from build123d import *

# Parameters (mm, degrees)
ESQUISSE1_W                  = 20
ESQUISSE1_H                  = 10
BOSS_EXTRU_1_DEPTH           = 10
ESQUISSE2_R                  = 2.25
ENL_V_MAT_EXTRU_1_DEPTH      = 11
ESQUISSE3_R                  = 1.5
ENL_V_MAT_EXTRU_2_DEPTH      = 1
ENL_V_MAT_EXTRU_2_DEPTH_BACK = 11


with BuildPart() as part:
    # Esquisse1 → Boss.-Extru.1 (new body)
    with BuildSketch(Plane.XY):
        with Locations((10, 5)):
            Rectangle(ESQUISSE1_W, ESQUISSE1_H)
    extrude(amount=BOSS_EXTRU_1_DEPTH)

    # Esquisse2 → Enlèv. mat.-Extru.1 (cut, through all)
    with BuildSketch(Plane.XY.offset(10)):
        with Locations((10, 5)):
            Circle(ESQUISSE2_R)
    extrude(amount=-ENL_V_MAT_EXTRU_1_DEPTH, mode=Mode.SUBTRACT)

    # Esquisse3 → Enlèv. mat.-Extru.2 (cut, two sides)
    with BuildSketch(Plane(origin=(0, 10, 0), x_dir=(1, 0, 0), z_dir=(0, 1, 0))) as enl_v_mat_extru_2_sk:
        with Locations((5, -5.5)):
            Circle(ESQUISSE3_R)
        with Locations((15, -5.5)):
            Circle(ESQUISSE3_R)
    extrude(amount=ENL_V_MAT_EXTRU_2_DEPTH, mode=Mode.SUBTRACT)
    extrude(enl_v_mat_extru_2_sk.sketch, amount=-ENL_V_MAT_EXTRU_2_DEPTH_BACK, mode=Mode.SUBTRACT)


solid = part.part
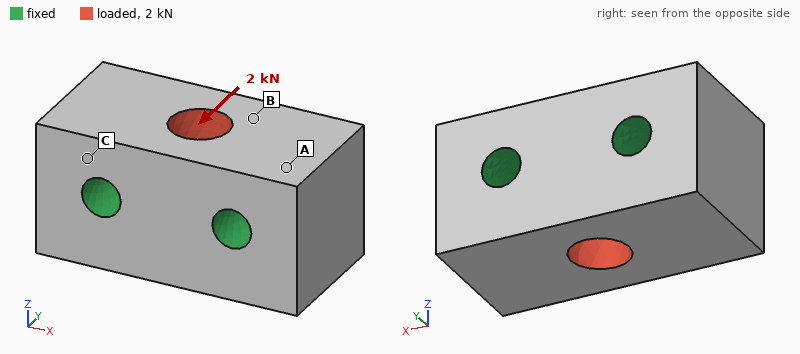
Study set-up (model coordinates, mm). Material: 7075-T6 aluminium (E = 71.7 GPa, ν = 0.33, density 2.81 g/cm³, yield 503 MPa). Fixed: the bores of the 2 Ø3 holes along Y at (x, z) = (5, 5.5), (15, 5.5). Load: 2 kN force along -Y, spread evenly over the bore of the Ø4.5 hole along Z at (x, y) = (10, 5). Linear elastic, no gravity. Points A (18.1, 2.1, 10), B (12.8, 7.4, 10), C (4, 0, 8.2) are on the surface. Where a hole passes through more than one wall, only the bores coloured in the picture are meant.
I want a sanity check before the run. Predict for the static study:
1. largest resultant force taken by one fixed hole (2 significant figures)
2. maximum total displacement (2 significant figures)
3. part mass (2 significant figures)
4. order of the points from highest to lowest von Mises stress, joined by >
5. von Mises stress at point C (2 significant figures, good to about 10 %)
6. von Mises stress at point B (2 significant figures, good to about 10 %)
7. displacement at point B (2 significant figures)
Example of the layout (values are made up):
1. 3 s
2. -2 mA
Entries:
1. 1.0 kN
2. 2.7 µm
3. 4.8 g
4. B > C > A
5. 7.0 MPa
6. 14 MPa
7. 1.0 µm
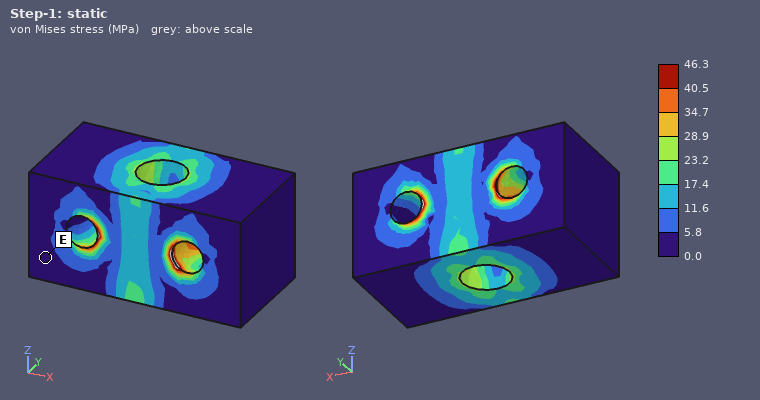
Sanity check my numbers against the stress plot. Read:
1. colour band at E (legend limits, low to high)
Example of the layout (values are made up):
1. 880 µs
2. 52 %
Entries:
1. 0.0 to 5.8 MPa
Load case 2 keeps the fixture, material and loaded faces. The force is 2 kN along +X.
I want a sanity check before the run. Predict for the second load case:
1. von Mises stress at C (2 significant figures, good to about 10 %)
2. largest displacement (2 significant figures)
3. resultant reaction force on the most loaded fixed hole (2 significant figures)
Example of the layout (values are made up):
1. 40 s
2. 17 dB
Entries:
1. 4.8 MPa
2. 1.4 µm
3. 1.0 kN
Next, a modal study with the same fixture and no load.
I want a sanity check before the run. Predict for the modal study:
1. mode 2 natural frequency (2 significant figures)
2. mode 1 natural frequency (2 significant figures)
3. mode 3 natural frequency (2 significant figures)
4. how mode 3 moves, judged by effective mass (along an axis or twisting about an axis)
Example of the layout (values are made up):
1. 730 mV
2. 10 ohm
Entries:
1. 100 kHz
2. 96 kHz
3. 110 kHz
4. along Y
